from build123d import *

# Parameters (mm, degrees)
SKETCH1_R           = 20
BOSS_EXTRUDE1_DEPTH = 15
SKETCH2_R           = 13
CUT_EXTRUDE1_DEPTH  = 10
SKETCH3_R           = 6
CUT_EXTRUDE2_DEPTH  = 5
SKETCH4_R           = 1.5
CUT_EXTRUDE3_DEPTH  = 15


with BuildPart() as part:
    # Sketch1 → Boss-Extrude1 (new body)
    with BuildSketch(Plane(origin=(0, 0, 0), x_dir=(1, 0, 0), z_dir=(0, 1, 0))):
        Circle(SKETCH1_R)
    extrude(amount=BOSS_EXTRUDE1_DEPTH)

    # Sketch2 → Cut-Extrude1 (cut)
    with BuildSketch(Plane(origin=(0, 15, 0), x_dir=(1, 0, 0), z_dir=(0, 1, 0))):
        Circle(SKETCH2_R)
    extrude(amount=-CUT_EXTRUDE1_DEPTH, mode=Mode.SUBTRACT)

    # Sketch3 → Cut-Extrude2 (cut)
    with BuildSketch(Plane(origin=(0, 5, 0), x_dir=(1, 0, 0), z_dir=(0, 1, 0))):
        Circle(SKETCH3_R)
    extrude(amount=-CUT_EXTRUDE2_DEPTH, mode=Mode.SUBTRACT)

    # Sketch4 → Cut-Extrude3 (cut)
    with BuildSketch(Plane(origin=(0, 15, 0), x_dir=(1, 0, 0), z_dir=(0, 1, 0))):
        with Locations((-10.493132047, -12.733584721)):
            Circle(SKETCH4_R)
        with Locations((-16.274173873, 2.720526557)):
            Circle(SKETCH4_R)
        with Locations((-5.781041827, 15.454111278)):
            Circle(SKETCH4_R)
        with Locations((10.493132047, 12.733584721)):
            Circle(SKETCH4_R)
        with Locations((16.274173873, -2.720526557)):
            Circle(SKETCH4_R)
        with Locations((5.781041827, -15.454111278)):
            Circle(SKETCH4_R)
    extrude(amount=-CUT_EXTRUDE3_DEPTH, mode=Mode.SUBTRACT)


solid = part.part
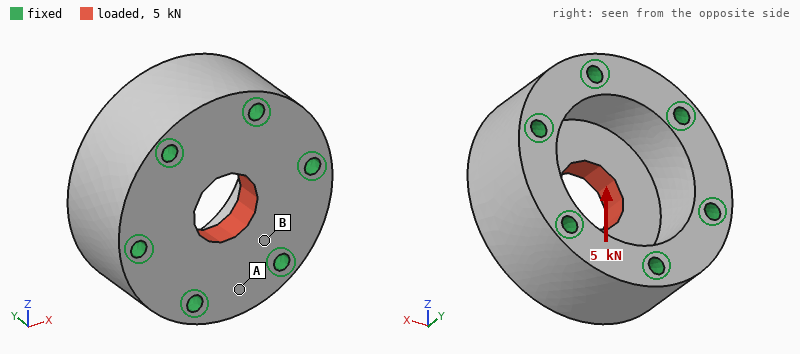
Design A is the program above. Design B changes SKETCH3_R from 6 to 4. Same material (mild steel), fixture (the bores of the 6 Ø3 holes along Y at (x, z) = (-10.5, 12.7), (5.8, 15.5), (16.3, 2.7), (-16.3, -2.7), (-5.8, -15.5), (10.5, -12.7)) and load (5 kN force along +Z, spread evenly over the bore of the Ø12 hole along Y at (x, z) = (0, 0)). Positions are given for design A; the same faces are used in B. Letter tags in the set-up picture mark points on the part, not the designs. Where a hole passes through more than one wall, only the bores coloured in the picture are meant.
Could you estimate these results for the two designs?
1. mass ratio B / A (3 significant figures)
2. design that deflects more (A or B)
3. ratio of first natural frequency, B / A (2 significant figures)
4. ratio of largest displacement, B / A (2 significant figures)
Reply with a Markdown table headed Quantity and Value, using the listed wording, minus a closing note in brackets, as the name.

| Quantity | Value |
|---|---|
| mass ratio B / A | 1.03 |
| design that deflects more | B |
| ratio of first natural frequency, B / A | 0.85 |
| ratio of largest displacement, B / A | 1.3 |
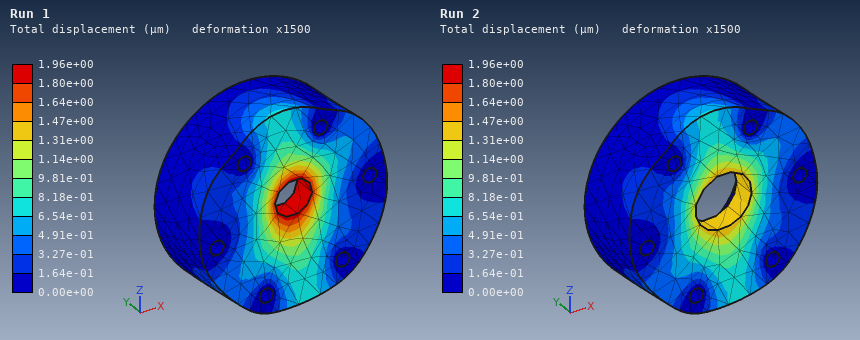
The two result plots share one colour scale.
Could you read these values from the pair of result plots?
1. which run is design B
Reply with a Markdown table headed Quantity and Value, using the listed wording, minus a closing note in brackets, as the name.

| Quantity | Value |
|---|---|
| which run is design B | Run 1 |
